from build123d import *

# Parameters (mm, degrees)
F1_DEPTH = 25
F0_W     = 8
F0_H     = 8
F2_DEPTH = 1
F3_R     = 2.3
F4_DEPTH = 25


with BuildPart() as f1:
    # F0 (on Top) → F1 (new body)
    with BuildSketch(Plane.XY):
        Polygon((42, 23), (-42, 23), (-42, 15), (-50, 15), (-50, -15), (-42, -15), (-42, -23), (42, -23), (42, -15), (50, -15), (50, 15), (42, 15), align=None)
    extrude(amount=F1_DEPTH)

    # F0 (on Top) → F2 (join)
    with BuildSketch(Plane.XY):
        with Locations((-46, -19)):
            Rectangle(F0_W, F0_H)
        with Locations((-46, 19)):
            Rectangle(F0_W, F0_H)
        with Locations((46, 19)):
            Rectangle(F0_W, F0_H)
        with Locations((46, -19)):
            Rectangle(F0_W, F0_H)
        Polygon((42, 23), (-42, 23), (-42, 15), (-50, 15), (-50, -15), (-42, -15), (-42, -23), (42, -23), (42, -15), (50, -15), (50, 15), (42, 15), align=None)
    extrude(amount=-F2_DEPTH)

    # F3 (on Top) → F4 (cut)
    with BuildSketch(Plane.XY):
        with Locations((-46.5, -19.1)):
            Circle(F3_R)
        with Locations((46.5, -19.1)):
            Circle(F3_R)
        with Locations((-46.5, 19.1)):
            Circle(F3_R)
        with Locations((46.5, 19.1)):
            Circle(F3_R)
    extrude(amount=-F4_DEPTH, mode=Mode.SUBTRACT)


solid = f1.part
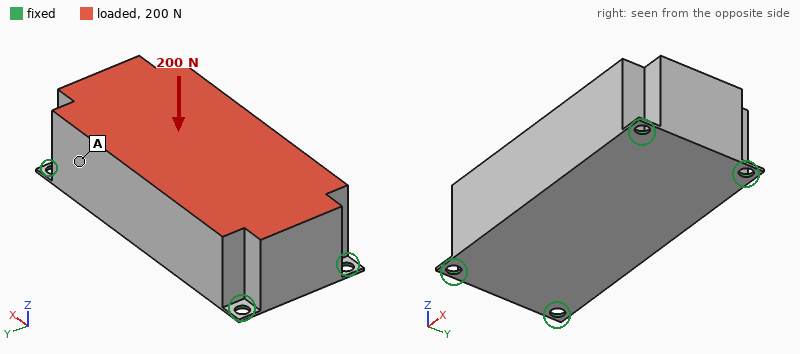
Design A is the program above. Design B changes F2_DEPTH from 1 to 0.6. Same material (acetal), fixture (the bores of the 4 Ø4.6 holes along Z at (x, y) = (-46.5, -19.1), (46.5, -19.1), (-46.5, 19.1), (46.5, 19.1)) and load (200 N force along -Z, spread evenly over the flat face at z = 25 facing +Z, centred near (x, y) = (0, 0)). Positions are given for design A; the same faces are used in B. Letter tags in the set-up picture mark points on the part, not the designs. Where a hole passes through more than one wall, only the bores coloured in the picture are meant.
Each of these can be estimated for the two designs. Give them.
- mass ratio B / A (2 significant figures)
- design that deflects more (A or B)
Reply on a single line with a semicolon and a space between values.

0.98; B
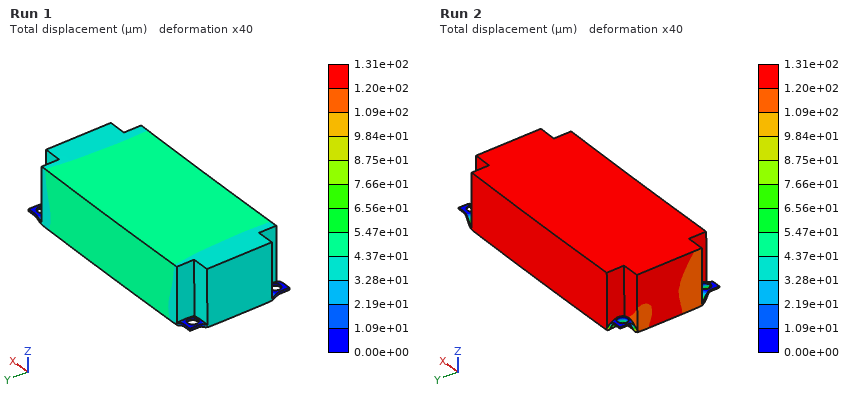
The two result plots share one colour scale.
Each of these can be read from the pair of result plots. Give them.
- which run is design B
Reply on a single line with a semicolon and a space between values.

Run 2
